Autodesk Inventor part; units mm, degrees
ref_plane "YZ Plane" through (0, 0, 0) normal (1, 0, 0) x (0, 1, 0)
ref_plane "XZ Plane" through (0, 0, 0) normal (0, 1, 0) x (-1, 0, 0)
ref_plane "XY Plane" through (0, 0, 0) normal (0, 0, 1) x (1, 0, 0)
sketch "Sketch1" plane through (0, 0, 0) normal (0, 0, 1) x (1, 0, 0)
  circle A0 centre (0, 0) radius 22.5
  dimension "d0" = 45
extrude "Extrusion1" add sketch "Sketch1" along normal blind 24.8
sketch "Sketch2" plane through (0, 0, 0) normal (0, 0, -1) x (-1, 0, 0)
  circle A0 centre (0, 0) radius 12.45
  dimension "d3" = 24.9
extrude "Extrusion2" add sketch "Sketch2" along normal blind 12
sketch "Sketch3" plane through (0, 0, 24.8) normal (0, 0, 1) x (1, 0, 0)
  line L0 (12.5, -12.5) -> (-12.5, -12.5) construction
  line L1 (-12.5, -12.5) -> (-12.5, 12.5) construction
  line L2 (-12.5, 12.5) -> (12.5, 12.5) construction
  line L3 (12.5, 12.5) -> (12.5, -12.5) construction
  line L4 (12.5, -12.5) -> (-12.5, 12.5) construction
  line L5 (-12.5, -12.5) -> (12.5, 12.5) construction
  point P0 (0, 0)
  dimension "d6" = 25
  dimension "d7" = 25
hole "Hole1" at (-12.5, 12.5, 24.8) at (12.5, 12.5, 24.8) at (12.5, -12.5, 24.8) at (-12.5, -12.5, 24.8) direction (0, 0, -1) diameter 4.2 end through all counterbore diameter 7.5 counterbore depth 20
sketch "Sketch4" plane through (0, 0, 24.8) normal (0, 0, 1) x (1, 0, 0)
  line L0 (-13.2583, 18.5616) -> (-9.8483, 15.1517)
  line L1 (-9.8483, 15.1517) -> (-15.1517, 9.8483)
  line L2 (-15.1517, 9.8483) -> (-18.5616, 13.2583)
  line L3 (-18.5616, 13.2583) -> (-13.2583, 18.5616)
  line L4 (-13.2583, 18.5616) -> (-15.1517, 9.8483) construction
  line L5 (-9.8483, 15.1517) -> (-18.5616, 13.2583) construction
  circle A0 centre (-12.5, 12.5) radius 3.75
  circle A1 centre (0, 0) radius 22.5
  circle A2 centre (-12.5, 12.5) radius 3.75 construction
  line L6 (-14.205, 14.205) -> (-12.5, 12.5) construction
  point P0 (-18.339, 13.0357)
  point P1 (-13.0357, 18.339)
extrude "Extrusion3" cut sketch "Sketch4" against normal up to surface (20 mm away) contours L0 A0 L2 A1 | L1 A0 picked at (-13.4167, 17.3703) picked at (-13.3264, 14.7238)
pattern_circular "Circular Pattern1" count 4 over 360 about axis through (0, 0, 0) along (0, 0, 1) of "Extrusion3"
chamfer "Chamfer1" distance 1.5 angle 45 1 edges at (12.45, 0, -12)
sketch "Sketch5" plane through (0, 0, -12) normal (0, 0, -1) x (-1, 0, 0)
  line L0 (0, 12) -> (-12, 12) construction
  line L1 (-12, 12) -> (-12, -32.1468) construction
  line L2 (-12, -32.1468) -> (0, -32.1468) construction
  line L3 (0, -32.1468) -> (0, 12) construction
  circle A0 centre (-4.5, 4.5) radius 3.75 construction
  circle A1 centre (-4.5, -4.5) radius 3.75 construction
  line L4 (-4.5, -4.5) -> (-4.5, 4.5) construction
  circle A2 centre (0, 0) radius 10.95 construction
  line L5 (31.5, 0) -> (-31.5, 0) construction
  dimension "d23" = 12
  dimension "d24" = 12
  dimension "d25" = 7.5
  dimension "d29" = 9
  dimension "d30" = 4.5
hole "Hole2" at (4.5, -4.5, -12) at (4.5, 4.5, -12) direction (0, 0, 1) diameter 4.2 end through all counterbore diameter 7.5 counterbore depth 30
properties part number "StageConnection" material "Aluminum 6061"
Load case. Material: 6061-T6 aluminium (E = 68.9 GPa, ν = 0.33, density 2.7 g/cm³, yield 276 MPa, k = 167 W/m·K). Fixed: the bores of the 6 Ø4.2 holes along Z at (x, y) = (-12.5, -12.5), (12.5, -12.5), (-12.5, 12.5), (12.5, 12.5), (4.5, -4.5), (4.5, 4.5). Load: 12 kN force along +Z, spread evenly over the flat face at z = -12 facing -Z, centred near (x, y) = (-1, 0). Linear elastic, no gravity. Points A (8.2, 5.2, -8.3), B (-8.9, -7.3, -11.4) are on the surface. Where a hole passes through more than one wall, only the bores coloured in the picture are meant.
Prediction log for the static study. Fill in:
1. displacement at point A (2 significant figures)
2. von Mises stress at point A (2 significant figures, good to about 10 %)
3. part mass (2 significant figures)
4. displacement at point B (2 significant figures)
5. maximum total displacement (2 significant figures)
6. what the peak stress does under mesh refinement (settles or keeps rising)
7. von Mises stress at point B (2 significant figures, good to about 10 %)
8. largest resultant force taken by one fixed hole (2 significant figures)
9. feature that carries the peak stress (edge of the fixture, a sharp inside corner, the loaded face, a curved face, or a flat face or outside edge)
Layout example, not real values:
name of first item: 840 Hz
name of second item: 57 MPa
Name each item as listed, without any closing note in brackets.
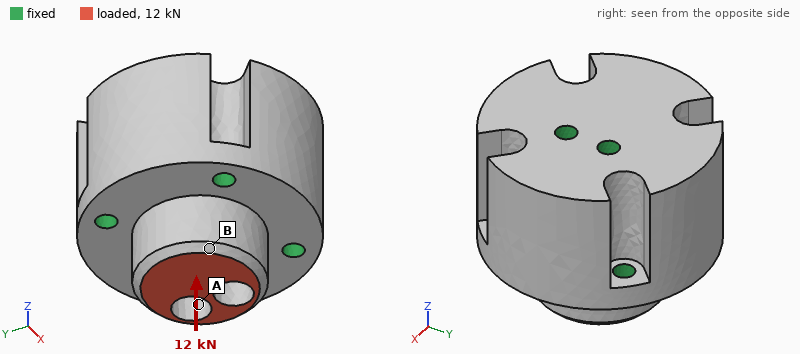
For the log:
displacement at point A: 8.8 µm
von Mises stress at point A: 39 MPa
part mass: 100 g
displacement at point B: 12 µm
maximum total displacement: 14 µm
what the peak stress does under mesh refinement: keeps rising
von Mises stress at point B: 17 MPa
largest resultant force taken by one fixed hole: 2.3 kN
feature that carries the peak stress: edge of the fixture
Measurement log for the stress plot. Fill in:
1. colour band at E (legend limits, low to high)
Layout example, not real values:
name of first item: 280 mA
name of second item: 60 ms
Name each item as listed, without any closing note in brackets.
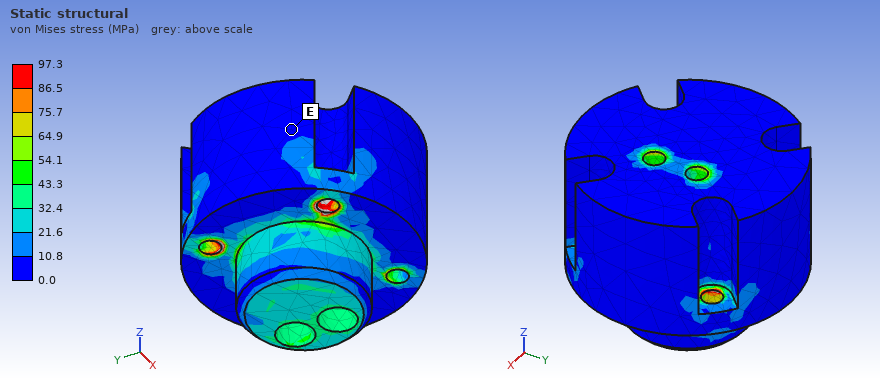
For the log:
colour band at E: 0.0 to 10.8 MPa
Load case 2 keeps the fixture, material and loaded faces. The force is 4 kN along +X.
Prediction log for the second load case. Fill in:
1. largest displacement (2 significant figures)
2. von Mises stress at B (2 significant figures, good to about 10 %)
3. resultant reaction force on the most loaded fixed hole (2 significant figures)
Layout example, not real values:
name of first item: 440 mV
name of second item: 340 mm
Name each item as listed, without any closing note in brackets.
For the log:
largest displacement: 19 µm
von Mises stress at B: 18 MPa
resultant reaction force on the most loaded fixed hole: 1.6 kN
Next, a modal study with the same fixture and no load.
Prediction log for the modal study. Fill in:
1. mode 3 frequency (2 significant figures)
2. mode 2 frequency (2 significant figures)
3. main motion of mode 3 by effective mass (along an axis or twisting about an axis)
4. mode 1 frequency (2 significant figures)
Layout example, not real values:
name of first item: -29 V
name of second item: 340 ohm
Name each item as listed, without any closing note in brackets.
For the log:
mode 3 frequency: 27 kHz
mode 2 frequency: 24 kHz
main motion of mode 3 by effective mass: along Y
mode 1 frequency: 24 kHz
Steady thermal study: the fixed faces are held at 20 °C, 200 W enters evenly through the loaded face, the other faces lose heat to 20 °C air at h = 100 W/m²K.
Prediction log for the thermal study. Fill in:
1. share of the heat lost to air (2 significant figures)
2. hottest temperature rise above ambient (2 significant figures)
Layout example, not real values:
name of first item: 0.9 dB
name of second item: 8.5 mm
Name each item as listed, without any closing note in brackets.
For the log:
share of the heat lost to air: 5.8 %
hottest temperature rise above ambient: 65 K
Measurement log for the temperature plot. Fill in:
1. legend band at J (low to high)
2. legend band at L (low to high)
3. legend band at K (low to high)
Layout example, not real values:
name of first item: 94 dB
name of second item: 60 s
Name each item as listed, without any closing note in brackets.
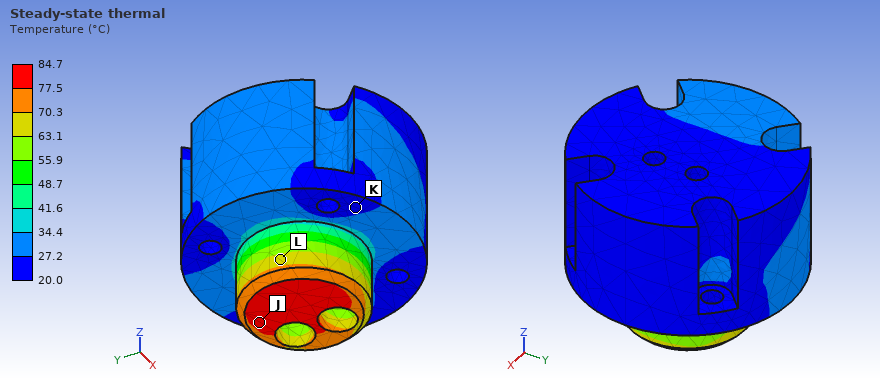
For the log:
legend band at J: 77.5 to 84.7 °C
legend band at L: 63.1 to 70.3 °C
legend band at K: 20.0 to 27.2 °C
